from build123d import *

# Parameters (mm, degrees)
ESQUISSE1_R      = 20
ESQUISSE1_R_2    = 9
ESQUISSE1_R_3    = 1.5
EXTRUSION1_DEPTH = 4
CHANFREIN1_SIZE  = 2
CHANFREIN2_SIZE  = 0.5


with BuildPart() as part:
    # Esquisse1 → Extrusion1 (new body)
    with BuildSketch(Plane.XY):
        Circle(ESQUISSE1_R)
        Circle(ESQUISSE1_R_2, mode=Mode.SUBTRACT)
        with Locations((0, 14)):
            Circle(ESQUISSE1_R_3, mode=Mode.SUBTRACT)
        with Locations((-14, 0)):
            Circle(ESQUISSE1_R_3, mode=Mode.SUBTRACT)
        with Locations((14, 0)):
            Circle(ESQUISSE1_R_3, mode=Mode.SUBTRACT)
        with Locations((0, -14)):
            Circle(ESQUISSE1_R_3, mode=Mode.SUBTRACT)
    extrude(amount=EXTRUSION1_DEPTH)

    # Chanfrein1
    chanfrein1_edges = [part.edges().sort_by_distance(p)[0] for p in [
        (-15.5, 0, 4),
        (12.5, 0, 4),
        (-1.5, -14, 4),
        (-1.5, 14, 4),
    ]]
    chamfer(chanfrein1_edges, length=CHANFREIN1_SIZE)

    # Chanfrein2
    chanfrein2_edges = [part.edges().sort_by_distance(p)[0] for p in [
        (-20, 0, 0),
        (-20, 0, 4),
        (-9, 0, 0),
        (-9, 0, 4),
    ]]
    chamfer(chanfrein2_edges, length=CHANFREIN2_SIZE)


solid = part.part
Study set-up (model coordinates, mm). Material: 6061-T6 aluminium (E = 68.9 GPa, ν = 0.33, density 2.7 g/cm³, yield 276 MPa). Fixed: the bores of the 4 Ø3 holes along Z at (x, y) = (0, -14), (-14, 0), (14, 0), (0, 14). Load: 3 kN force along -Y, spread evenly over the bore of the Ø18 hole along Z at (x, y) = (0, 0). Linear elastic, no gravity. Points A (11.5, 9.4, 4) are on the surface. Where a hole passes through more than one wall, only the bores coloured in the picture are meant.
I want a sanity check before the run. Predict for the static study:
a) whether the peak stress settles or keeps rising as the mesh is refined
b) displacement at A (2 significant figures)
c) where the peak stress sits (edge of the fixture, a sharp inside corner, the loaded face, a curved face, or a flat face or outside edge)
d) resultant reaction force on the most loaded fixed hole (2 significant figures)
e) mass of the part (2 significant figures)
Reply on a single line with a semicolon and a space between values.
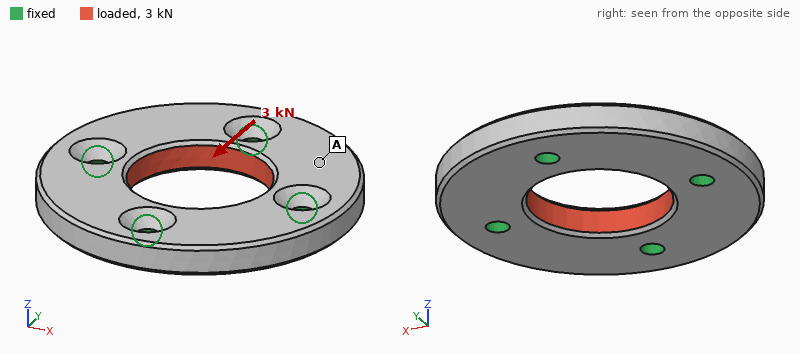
keeps rising; 3.7 µm; edge of the fixture; 760 N; 10 g
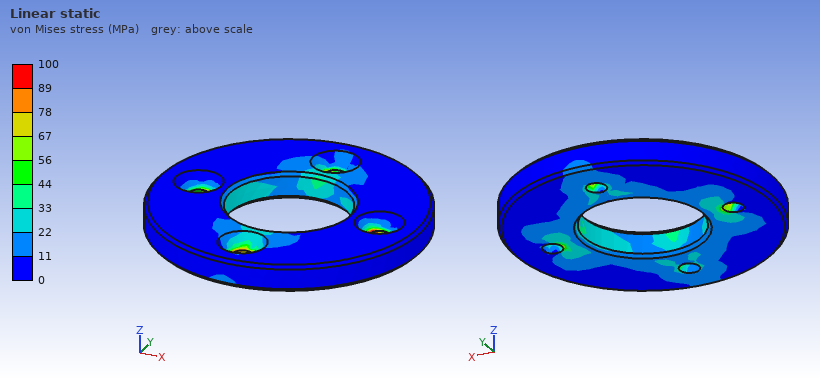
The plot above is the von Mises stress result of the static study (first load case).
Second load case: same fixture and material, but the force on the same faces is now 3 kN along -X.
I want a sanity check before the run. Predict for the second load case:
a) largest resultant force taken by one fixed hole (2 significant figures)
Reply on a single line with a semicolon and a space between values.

760 N
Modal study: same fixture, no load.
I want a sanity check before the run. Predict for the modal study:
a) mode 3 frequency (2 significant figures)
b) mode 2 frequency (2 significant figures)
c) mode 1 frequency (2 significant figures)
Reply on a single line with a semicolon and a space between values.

21 kHz; 21 kHz; 18 kHz
